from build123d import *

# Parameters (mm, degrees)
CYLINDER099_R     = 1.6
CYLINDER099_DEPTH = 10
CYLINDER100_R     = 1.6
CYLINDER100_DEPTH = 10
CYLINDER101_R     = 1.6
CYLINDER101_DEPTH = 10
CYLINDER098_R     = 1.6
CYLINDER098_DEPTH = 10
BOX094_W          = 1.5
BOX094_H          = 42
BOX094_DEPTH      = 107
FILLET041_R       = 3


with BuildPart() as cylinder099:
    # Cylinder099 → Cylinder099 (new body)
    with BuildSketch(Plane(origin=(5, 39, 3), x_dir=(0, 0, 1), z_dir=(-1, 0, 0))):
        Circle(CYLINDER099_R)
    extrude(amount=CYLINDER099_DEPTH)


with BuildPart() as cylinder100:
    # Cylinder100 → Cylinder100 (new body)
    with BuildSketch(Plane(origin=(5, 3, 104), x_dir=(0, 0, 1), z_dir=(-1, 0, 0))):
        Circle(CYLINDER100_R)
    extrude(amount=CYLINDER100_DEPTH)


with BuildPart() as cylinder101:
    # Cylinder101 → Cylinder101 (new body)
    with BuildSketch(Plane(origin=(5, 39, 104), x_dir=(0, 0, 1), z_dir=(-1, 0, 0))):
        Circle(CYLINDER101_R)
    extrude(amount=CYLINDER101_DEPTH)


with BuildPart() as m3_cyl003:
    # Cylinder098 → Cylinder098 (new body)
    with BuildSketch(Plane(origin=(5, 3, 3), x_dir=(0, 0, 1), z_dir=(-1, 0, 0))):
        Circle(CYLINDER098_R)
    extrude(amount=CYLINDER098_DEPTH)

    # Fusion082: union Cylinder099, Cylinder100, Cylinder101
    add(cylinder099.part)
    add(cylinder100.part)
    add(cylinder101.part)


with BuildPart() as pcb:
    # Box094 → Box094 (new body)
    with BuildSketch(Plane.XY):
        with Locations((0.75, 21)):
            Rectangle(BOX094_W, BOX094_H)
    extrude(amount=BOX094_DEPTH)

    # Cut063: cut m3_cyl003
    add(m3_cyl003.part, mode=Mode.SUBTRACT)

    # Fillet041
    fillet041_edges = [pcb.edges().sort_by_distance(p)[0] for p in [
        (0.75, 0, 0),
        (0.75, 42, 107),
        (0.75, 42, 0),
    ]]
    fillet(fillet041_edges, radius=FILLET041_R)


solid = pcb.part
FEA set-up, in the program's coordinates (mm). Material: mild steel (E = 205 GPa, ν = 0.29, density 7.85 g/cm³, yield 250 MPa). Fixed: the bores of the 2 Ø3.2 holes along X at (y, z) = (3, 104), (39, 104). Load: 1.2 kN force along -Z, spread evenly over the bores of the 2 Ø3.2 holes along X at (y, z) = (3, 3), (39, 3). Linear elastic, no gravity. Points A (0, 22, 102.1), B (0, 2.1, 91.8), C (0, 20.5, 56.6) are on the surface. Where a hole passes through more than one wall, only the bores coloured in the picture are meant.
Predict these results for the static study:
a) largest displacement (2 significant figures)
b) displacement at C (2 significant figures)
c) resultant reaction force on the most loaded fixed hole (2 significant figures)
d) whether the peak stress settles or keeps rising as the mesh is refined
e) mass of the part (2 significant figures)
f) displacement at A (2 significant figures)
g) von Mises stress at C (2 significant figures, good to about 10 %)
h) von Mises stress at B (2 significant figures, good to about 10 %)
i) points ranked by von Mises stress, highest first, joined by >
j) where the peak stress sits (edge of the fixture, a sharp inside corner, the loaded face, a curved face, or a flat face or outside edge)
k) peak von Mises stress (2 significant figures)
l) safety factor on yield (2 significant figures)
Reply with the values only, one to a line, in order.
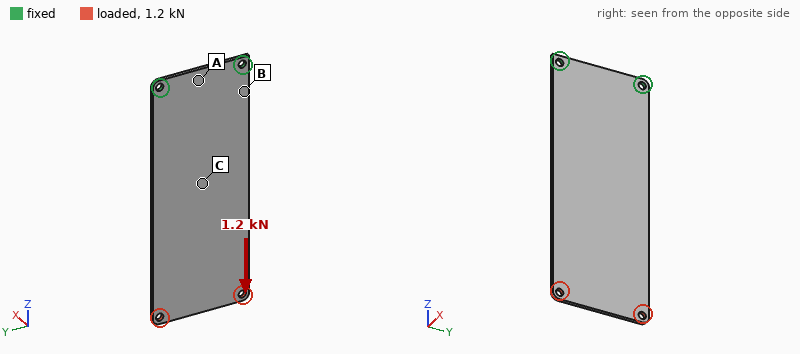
15 µm
5.9 µm
630 N
settles
52 g
3.1 µm
19 MPa
31 MPa
B > C > A
the loaded face
190 MPa
1.3
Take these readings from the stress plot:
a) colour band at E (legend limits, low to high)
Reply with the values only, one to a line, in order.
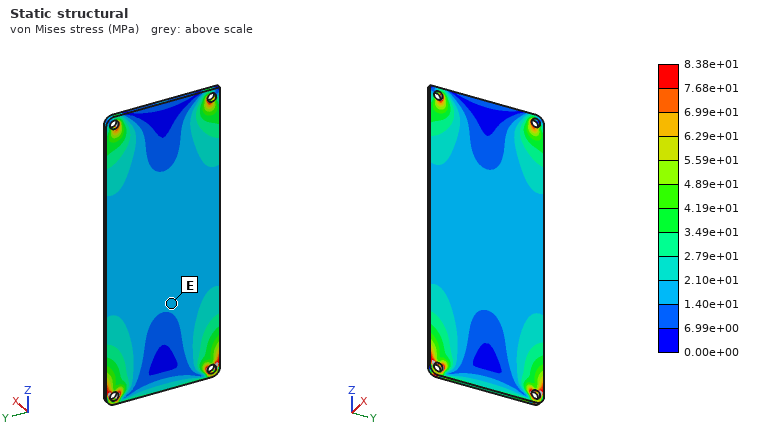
1.40e+01 to 2.10e+01 MPa
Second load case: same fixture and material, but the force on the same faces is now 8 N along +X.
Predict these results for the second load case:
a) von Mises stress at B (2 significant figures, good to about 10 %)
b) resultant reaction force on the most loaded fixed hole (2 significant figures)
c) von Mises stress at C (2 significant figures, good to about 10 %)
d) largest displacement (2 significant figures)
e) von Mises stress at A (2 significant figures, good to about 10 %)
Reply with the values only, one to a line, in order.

51 MPa
4.0 N
27 MPa
1.3 mm
16 MPa
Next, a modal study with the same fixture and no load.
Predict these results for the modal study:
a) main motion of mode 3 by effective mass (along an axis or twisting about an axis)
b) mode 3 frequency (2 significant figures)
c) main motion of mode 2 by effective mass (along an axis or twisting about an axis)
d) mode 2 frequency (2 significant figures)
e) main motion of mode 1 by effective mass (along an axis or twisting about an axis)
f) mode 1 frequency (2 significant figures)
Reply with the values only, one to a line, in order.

along X
690 Hz
twisting about Z
610 Hz
along X
110 Hz
